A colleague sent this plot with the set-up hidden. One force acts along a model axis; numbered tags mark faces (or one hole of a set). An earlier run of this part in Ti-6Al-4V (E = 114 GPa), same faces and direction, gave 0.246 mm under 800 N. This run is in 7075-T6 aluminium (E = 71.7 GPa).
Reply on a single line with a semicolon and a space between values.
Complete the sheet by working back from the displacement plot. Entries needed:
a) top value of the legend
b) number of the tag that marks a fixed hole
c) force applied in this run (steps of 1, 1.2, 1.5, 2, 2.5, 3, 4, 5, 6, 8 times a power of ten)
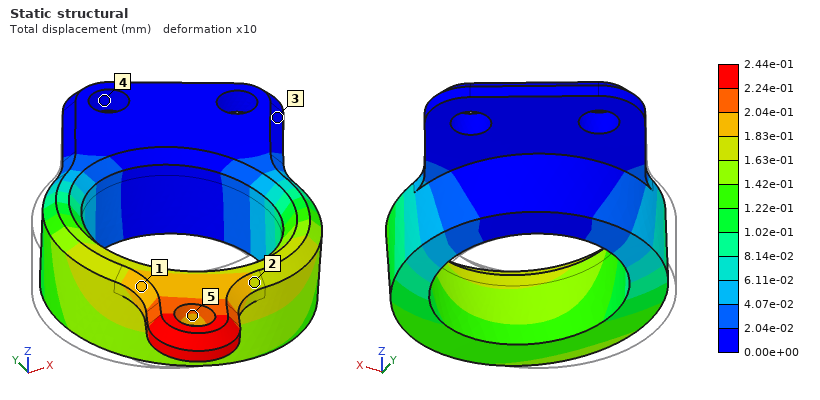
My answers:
2.44e-01 mm; 4; 500 N
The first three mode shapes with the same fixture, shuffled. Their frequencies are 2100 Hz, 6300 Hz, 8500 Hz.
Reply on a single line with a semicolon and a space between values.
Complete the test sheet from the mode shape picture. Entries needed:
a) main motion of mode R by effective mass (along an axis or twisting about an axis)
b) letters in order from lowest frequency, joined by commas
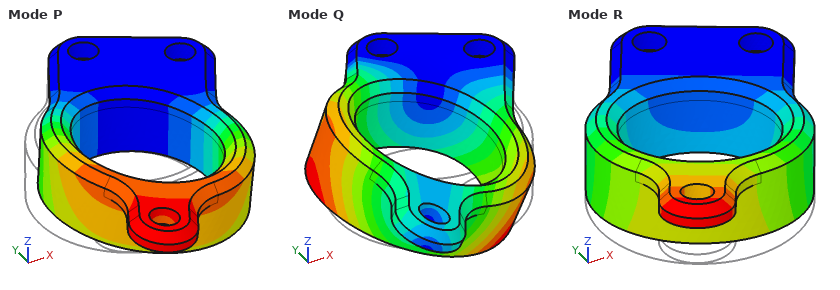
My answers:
along Z; R, P, Q
